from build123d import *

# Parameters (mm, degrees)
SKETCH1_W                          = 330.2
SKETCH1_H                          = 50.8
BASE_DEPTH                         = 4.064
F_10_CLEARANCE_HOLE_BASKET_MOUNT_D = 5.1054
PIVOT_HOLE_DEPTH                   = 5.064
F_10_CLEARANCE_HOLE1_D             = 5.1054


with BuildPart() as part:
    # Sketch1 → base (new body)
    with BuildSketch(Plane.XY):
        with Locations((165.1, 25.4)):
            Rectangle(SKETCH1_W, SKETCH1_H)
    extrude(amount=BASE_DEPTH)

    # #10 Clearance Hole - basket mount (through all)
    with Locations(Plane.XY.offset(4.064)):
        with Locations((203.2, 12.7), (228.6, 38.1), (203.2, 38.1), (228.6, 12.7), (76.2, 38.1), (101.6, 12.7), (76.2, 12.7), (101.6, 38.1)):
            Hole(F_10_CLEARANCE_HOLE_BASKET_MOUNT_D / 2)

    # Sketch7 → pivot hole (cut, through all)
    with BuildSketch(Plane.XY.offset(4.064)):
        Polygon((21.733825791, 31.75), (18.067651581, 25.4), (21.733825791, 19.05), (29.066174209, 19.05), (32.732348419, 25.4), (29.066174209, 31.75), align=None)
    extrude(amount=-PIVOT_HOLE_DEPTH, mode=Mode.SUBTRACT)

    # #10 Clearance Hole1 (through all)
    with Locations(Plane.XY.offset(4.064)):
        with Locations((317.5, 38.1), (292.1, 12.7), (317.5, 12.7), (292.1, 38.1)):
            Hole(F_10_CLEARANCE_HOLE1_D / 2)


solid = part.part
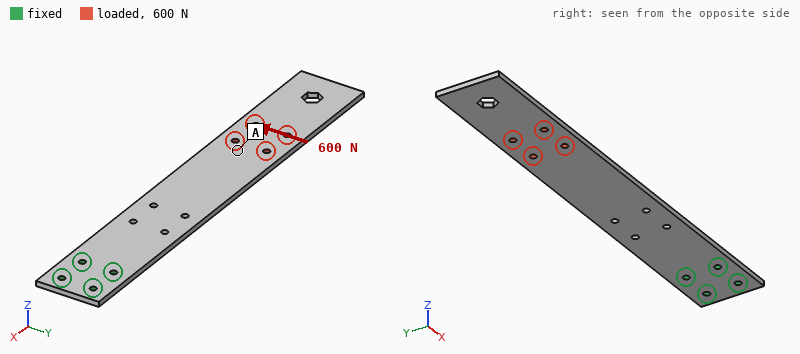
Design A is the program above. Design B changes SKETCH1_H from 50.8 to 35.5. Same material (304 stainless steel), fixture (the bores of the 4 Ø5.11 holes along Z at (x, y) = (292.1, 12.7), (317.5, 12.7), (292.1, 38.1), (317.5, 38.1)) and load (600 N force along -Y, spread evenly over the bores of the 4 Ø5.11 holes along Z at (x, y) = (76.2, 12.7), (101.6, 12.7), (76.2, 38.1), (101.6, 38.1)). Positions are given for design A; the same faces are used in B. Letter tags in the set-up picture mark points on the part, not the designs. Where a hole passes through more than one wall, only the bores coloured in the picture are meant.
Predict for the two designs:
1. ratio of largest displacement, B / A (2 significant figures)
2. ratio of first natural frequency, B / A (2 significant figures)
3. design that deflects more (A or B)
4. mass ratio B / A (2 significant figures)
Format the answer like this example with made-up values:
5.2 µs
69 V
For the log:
2.8
1.0
B
0.69
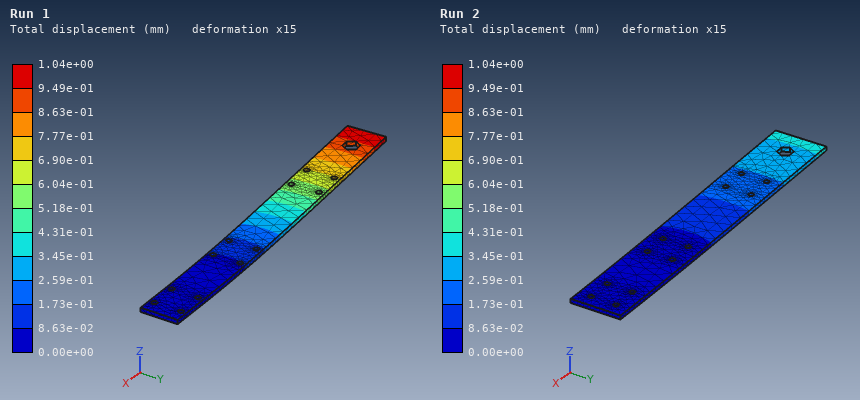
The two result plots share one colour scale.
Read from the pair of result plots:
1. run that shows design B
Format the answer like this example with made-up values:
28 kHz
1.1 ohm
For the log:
Run 1
